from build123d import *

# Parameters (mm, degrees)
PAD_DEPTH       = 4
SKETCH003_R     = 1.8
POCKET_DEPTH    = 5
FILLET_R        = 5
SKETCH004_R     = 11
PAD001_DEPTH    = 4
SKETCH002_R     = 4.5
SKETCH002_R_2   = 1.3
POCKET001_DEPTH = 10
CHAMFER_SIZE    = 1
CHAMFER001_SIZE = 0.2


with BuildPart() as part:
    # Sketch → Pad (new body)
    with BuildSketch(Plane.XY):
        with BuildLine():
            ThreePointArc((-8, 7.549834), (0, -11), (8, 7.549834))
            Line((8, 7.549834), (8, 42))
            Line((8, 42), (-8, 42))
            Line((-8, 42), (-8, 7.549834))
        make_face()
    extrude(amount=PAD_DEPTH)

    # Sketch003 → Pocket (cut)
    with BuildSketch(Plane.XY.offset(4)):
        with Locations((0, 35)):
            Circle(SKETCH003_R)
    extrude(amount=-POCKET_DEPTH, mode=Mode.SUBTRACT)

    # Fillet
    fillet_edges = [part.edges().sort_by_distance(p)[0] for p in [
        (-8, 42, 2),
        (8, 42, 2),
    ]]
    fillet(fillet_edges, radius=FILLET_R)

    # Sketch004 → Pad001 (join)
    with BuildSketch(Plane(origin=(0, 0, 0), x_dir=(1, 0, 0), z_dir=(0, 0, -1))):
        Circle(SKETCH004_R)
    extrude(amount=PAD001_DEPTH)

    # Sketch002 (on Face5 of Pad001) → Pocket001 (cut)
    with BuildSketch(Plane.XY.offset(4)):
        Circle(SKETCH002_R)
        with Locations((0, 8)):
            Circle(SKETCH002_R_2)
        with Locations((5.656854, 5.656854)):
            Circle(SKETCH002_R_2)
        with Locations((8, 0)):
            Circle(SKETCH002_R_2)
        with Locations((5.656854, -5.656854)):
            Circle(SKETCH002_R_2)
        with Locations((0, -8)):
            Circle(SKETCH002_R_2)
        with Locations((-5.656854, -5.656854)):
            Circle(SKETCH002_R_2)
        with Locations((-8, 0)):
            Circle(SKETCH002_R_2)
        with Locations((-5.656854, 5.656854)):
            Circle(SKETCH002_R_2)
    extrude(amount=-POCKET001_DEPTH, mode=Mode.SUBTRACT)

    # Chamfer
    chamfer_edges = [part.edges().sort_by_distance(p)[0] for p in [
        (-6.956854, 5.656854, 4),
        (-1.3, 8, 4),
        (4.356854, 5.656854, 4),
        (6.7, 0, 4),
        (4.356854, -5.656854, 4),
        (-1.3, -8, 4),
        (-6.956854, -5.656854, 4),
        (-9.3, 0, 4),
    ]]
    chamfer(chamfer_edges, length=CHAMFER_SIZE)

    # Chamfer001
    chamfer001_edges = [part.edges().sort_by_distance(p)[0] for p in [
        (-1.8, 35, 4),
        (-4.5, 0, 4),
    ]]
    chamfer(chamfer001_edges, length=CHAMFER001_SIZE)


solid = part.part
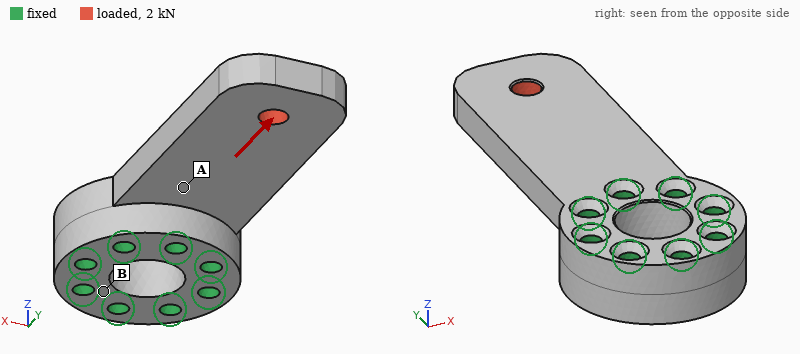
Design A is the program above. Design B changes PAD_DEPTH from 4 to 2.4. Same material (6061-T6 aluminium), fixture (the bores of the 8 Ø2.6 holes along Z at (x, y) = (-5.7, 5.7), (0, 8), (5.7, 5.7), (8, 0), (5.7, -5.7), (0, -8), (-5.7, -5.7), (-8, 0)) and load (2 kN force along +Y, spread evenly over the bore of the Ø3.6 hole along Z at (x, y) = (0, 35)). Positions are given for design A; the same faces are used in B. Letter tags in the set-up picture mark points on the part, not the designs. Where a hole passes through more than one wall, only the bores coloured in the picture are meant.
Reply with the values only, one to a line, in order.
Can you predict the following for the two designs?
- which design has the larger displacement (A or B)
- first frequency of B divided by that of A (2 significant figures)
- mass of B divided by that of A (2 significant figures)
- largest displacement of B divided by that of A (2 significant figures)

B
0.63
0.70
3.2
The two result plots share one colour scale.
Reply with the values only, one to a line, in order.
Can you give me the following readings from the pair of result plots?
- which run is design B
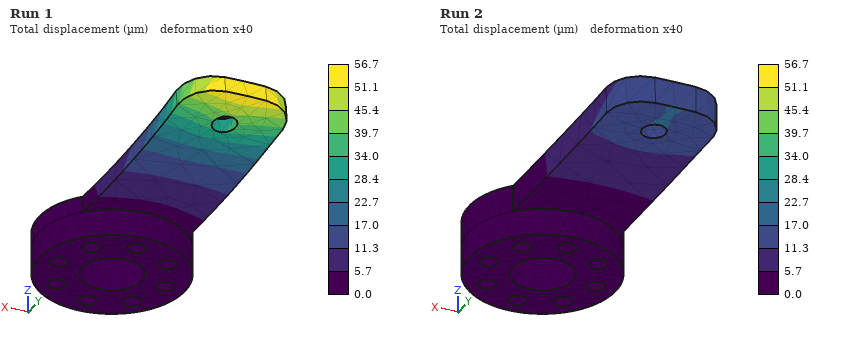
Run 1
